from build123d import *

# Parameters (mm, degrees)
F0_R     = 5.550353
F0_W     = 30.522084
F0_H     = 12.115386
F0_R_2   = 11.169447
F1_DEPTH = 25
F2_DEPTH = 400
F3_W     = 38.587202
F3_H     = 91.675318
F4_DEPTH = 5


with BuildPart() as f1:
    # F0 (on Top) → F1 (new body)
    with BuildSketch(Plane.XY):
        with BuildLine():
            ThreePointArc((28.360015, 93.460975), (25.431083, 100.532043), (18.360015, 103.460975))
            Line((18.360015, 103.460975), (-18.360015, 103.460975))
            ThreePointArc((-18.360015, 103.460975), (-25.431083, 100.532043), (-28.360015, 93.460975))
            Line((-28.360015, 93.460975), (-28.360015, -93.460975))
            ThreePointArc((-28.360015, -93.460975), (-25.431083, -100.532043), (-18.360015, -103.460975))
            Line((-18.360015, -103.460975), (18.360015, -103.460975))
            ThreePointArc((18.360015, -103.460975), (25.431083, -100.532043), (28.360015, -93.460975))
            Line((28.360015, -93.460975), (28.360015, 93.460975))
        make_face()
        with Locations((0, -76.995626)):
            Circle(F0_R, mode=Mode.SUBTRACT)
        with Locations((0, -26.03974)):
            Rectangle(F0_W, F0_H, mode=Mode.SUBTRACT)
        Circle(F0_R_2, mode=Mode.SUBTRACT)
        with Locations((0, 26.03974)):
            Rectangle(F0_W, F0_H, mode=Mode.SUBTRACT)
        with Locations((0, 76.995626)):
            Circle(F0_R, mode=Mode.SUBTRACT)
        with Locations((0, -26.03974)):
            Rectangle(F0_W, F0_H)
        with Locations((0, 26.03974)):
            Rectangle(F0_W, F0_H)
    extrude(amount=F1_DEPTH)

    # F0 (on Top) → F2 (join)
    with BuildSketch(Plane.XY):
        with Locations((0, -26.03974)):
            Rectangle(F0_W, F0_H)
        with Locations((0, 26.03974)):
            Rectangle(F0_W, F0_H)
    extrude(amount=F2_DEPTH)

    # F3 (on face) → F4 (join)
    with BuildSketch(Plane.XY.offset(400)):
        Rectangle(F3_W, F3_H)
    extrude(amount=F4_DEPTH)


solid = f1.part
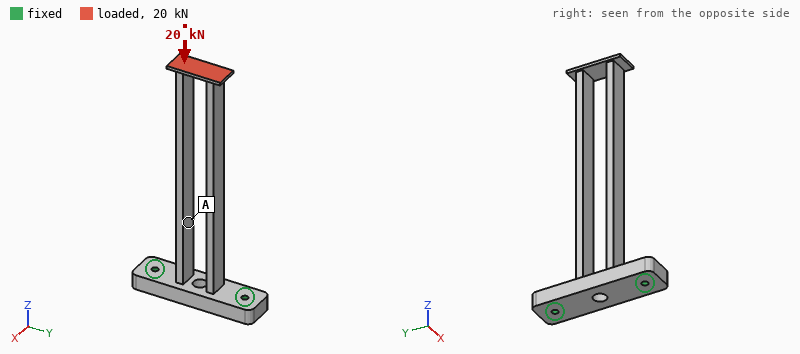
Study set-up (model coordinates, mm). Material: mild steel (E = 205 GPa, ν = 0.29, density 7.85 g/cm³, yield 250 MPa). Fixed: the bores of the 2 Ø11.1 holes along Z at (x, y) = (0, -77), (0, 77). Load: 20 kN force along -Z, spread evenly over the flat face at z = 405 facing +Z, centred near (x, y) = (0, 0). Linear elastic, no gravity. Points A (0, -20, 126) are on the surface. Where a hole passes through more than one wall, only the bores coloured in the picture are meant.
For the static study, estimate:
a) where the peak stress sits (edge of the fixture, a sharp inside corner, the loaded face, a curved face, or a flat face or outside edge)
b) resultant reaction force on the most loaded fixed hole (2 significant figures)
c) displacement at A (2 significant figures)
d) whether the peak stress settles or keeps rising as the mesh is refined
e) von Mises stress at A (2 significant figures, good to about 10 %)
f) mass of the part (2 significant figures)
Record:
edge of the fixture
10 kN
0.036 mm
keeps rising
23 MPa
4.5 kg
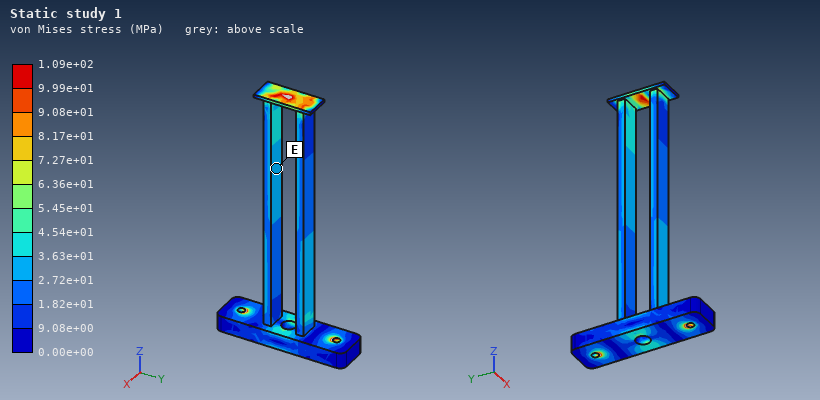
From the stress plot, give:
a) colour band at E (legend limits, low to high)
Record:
2.72e+01 to 3.63e+01 MPa
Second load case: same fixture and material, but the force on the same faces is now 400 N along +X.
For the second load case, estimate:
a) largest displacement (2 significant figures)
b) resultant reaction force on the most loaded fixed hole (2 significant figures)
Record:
0.74 mm
200 N
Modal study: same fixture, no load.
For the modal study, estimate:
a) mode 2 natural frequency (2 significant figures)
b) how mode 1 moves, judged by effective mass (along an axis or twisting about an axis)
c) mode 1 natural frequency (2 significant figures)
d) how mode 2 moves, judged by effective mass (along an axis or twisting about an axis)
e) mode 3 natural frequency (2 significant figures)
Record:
140 Hz
along Y
93 Hz
along X
330 Hz
